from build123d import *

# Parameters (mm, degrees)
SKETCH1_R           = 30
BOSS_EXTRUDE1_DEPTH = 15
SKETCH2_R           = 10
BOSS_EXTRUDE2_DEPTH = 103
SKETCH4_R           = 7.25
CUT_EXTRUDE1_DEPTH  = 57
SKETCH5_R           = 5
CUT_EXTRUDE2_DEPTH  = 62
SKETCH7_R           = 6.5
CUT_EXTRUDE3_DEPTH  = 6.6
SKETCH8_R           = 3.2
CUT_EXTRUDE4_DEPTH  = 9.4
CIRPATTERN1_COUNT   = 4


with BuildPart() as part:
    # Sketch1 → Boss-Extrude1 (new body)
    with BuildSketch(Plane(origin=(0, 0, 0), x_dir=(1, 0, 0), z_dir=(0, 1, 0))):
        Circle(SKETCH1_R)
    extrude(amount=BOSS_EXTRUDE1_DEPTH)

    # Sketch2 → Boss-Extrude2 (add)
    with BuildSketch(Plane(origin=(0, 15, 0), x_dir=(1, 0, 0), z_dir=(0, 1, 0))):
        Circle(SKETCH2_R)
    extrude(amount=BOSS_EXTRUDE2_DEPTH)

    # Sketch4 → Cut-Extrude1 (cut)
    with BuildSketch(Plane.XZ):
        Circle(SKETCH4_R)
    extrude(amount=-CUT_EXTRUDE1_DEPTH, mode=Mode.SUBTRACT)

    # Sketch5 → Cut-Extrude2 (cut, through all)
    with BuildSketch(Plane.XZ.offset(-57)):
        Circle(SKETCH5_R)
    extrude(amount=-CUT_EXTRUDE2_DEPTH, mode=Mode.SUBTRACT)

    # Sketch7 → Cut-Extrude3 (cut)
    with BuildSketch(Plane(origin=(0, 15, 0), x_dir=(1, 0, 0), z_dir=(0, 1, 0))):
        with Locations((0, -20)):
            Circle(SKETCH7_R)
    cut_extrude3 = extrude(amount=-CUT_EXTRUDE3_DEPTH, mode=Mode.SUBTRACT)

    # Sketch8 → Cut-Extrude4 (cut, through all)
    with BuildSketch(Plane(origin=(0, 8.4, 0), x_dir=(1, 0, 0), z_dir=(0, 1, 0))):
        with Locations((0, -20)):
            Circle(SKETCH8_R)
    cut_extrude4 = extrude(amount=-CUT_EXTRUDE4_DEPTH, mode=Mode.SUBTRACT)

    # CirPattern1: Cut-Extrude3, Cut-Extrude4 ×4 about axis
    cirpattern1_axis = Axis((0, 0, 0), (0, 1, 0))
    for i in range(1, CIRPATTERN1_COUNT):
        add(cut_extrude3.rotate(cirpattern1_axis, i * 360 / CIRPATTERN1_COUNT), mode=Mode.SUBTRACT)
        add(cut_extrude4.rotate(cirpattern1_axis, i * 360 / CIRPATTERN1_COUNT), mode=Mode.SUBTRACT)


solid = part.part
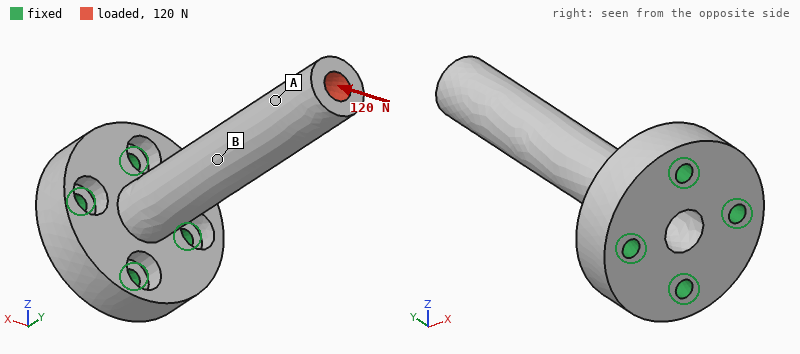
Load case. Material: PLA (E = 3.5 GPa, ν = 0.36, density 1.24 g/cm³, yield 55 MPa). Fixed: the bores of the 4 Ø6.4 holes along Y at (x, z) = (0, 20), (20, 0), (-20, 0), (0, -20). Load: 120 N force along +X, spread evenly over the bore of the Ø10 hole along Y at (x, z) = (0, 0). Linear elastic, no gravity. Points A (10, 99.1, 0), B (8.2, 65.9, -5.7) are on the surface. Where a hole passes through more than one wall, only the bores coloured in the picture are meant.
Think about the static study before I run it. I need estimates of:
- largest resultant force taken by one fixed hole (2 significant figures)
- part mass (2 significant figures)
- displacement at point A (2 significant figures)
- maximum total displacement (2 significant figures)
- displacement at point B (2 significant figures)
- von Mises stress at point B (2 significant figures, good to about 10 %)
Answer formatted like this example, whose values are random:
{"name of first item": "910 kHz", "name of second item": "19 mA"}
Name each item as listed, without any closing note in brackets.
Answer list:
{"largest resultant force taken by one fixed hole": "270 N", "part mass": "69 g", "displacement at point A": "1.2 mm", "maximum total displacement": "1.6 mm", "displacement at point B": "0.62 mm", "von Mises stress at point B": "3.2 MPa"}
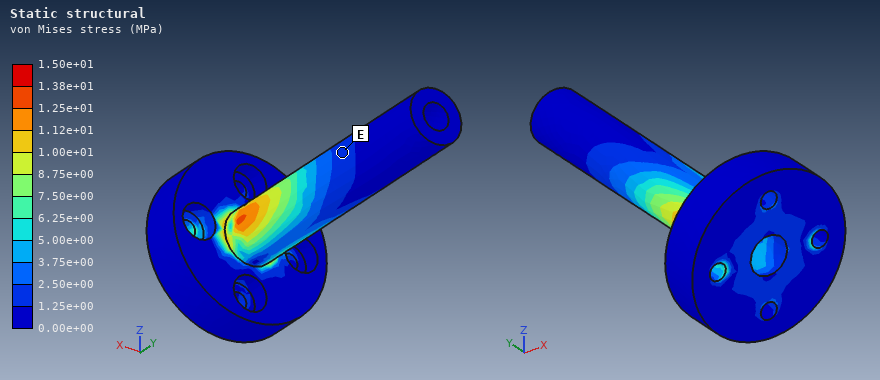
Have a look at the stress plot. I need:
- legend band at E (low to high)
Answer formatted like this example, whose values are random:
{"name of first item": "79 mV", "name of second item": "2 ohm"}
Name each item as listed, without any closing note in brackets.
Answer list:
{"legend band at E": "1.25e+00 to 2.50e+00 MPa"}
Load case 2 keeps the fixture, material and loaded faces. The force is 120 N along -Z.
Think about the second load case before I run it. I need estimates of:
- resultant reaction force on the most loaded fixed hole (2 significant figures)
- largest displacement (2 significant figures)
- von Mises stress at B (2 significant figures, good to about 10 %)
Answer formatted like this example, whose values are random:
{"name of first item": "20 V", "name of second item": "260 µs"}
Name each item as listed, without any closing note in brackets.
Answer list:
{"resultant reaction force on the most loaded fixed hole": "270 N", "largest displacement": "1.6 mm", "von Mises stress at B": "2.3 MPa"}
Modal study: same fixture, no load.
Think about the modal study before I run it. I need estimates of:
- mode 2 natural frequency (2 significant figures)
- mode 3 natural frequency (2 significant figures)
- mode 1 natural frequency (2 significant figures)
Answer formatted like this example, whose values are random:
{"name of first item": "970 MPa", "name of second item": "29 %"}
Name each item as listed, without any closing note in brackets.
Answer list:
{"mode 2 natural frequency": "390 Hz", "mode 3 natural frequency": "2200 Hz", "mode 1 natural frequency": "390 Hz"}
